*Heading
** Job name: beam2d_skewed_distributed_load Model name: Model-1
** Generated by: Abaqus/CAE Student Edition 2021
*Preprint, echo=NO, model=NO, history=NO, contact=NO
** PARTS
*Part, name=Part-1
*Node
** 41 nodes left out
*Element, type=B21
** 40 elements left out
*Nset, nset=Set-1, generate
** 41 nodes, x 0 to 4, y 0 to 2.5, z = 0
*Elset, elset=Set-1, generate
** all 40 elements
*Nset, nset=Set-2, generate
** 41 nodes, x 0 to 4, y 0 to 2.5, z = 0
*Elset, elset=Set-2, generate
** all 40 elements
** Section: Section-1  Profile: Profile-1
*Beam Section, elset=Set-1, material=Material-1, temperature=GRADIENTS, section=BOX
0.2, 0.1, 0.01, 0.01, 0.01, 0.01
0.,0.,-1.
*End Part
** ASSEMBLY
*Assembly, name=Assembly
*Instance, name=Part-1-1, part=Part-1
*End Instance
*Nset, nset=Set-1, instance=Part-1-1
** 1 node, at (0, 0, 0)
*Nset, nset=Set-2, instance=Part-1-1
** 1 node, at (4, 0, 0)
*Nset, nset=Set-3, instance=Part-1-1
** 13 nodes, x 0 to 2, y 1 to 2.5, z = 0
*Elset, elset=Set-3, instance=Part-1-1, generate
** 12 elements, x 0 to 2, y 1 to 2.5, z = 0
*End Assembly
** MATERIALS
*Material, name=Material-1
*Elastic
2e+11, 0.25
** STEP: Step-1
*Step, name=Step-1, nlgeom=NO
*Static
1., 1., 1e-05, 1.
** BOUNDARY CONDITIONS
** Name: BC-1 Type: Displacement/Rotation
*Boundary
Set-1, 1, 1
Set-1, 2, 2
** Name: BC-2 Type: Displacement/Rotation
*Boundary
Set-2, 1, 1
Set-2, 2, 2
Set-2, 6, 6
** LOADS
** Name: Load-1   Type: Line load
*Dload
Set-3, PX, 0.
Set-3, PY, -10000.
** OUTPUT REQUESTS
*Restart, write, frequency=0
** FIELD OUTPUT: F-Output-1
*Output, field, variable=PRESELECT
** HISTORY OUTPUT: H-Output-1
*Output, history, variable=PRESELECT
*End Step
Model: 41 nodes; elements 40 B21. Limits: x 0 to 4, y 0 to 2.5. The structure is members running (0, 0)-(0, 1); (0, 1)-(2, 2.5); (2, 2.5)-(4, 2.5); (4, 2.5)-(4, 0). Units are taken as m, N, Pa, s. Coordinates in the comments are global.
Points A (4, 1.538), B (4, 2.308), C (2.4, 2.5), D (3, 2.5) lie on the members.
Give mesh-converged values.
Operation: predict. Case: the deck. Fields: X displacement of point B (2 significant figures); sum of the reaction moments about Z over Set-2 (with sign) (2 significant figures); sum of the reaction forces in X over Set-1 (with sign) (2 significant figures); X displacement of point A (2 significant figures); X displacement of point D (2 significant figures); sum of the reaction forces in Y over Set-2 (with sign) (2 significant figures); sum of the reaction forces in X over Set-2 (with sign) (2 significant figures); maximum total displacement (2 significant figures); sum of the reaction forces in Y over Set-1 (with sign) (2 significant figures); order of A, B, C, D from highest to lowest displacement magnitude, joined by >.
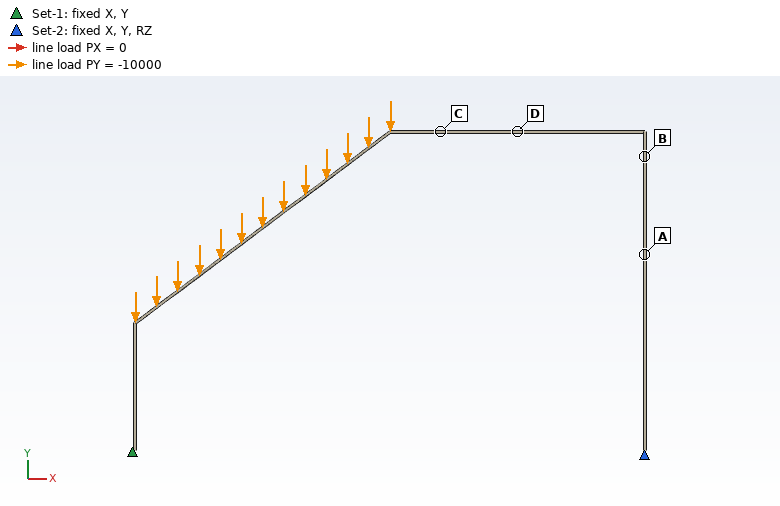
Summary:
0.0040 m
6600 N·m
5100 N
0.0026 m
0.0041 m
4600 N
-5100 N
0.0057 m
20000 N
C > D > B > A
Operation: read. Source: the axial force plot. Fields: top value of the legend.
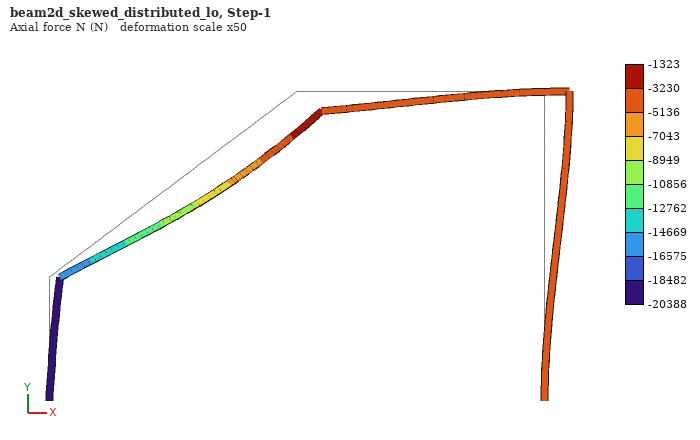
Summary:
-1323 N
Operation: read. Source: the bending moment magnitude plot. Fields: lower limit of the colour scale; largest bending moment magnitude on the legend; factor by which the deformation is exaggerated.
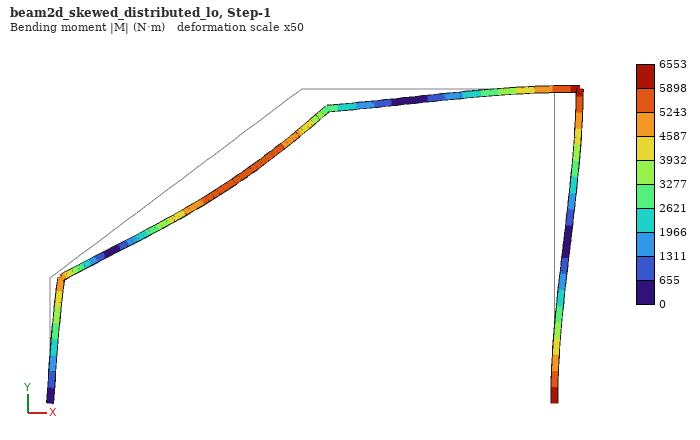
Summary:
0 N·m
6553 N·m
50
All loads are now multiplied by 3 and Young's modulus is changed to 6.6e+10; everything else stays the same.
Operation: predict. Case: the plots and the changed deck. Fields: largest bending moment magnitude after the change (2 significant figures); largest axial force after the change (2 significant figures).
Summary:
20000 N·m
-4000 N
